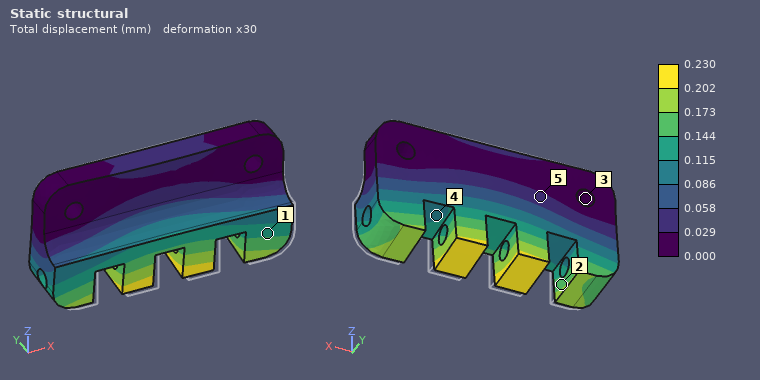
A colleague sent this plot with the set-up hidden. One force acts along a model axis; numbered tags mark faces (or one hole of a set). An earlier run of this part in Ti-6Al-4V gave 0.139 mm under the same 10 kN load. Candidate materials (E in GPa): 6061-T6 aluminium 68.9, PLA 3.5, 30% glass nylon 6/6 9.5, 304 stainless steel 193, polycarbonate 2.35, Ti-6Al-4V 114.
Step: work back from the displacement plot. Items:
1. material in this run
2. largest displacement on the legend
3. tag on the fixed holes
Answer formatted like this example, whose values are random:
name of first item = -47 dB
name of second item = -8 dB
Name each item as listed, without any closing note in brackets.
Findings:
material in this run = 6061-T6 aluminium
largest displacement on the legend = 0.230 mm
tag on the fixed holes = 3
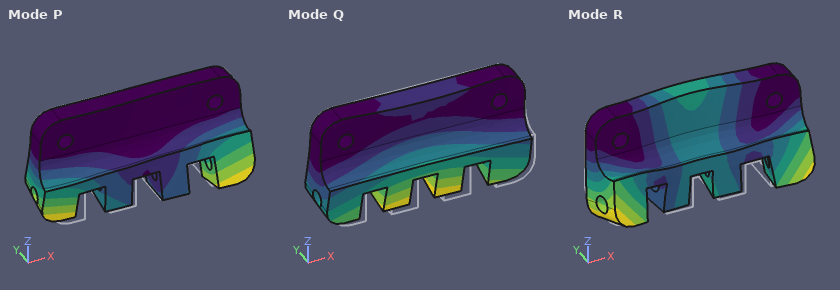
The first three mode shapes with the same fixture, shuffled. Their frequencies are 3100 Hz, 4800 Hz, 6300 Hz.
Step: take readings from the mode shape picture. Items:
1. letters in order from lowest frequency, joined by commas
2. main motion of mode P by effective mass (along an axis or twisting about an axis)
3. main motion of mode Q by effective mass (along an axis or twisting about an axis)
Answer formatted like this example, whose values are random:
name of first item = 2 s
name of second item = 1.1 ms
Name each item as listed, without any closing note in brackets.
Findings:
letters in order from lowest frequency, joined by commas = Q, P, R
main motion of mode P by effective mass = twisting about Z
main motion of mode Q by effective mass = along Y
